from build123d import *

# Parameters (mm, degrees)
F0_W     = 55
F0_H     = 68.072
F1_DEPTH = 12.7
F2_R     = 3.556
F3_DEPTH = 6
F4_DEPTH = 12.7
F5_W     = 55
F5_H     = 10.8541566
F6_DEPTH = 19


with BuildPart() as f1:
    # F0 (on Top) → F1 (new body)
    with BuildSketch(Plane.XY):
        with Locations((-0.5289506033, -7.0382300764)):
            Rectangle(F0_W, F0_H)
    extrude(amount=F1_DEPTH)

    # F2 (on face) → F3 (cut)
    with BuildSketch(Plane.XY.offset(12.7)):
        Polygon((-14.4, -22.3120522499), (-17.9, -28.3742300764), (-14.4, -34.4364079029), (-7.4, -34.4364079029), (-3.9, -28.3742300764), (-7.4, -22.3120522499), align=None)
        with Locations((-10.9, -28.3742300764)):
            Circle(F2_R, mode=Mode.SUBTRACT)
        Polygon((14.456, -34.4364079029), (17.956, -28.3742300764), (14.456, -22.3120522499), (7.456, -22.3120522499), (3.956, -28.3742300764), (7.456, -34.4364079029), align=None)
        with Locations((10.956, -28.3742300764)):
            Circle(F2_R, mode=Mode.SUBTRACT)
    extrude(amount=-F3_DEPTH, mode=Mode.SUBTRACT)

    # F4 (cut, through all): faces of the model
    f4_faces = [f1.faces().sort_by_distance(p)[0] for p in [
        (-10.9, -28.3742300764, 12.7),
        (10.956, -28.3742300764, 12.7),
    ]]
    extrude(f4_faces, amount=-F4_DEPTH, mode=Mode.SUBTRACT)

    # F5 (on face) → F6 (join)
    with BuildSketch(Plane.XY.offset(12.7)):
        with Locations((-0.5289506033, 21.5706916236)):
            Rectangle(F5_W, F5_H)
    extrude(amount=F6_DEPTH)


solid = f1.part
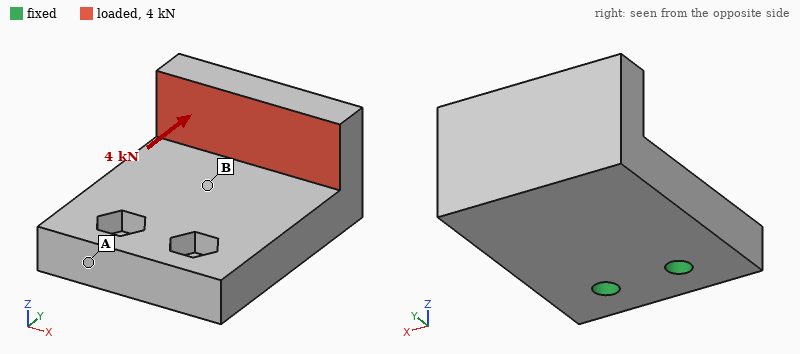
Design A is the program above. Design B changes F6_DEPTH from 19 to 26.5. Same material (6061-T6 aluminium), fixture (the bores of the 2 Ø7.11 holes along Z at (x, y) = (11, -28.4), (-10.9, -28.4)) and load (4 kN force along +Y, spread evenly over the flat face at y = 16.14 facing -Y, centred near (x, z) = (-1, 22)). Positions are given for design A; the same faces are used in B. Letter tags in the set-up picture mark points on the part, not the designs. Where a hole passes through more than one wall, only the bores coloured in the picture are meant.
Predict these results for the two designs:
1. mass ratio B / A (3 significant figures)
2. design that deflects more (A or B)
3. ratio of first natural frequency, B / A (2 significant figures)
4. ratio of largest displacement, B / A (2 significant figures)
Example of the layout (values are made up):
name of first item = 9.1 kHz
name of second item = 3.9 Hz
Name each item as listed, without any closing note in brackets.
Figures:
mass ratio B / A = 1.08
design that deflects more = B
ratio of first natural frequency, B / A = 0.89
ratio of largest displacement, B / A = 1.4
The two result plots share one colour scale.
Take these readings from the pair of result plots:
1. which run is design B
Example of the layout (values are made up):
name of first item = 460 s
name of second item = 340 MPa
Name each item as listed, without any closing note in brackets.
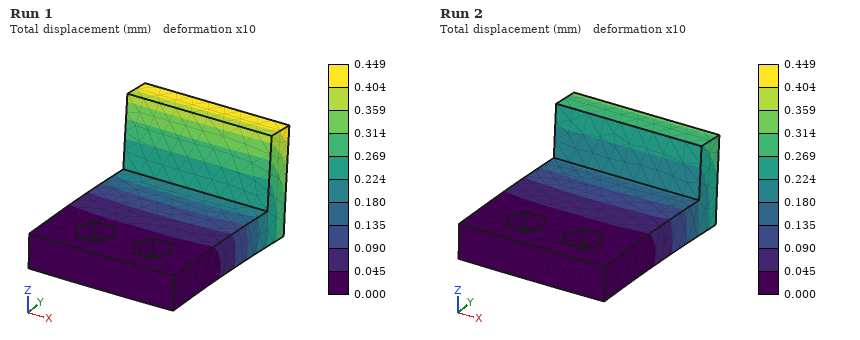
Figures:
which run is design B = Run 1
